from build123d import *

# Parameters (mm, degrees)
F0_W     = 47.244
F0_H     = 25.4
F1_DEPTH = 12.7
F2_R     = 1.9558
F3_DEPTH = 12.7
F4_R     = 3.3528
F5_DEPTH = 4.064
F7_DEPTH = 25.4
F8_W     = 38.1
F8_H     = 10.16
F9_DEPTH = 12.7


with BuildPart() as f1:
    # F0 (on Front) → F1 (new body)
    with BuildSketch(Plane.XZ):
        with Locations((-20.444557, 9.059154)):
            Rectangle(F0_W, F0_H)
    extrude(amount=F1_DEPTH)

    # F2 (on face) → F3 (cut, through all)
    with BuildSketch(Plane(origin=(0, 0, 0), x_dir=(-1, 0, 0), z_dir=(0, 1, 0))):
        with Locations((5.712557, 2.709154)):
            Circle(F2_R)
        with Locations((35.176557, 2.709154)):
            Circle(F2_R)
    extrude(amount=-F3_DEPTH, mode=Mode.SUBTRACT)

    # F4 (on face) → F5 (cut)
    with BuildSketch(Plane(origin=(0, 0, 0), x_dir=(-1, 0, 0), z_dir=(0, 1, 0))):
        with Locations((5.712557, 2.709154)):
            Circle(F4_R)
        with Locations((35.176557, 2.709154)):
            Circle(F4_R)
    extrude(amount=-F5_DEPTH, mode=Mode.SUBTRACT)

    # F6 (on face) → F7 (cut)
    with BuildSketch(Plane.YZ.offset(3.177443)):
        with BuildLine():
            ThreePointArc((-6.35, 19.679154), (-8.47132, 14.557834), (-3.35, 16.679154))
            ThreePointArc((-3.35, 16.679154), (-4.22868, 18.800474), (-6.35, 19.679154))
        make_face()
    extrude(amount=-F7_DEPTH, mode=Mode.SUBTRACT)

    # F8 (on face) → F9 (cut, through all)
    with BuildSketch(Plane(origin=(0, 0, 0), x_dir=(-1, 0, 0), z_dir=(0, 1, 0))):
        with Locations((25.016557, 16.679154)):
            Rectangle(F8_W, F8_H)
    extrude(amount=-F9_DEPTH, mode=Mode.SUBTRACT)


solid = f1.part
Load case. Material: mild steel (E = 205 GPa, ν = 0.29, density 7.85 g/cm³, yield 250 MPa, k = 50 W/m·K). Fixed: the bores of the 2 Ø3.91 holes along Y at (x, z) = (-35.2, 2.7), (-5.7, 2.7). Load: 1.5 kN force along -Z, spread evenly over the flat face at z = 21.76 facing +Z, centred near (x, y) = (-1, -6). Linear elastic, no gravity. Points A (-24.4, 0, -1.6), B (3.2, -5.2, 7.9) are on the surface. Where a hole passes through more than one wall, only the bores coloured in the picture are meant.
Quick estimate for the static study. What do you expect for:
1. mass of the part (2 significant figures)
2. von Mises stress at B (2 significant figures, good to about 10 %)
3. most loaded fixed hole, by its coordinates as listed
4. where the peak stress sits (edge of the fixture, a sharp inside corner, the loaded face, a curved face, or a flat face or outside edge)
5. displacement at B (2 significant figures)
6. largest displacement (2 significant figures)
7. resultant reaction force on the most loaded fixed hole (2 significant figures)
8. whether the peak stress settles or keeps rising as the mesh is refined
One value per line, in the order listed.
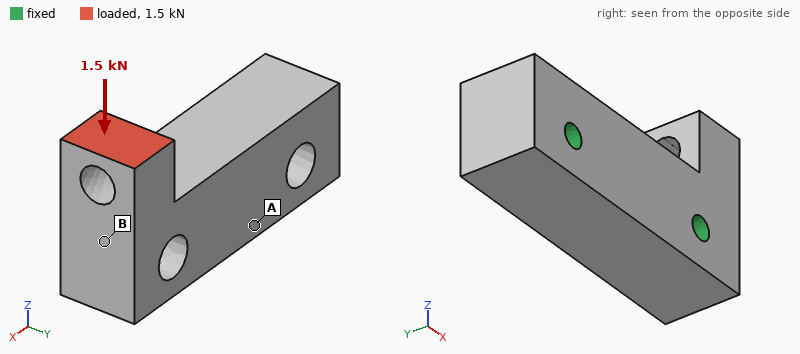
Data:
75 g
9.2 MPa
(-5.7, 2.7)
edge of the fixture
1.7 µm
4.8 µm
1.6 kN
keeps rising
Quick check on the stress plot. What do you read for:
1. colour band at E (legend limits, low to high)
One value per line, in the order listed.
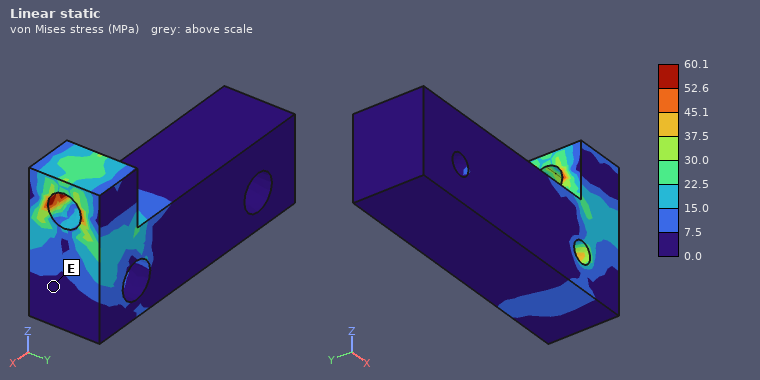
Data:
0.0 to 7.5 MPa
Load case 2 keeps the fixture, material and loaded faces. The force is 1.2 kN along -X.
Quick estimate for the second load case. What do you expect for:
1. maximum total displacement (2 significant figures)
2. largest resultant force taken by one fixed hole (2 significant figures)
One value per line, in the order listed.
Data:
19 µm
850 N
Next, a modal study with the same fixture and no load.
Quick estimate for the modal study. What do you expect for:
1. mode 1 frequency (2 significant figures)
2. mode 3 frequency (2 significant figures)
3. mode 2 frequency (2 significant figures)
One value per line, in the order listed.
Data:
19 kHz
31 kHz
22 kHz
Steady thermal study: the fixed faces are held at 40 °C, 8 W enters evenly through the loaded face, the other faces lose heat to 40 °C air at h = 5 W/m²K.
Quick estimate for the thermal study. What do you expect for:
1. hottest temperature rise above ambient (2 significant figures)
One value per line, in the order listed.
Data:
34 K
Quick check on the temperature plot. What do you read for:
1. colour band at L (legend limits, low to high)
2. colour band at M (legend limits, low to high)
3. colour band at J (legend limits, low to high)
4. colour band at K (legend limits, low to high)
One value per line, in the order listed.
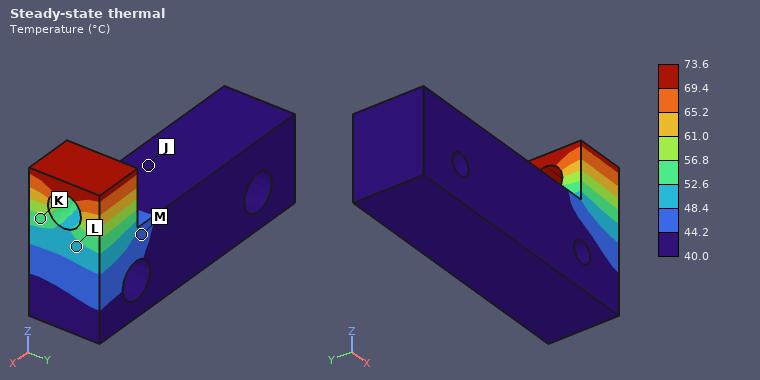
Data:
48.4 to 52.6 °C
44.2 to 48.4 °C
40.0 to 44.2 °C
52.6 to 56.8 °C
